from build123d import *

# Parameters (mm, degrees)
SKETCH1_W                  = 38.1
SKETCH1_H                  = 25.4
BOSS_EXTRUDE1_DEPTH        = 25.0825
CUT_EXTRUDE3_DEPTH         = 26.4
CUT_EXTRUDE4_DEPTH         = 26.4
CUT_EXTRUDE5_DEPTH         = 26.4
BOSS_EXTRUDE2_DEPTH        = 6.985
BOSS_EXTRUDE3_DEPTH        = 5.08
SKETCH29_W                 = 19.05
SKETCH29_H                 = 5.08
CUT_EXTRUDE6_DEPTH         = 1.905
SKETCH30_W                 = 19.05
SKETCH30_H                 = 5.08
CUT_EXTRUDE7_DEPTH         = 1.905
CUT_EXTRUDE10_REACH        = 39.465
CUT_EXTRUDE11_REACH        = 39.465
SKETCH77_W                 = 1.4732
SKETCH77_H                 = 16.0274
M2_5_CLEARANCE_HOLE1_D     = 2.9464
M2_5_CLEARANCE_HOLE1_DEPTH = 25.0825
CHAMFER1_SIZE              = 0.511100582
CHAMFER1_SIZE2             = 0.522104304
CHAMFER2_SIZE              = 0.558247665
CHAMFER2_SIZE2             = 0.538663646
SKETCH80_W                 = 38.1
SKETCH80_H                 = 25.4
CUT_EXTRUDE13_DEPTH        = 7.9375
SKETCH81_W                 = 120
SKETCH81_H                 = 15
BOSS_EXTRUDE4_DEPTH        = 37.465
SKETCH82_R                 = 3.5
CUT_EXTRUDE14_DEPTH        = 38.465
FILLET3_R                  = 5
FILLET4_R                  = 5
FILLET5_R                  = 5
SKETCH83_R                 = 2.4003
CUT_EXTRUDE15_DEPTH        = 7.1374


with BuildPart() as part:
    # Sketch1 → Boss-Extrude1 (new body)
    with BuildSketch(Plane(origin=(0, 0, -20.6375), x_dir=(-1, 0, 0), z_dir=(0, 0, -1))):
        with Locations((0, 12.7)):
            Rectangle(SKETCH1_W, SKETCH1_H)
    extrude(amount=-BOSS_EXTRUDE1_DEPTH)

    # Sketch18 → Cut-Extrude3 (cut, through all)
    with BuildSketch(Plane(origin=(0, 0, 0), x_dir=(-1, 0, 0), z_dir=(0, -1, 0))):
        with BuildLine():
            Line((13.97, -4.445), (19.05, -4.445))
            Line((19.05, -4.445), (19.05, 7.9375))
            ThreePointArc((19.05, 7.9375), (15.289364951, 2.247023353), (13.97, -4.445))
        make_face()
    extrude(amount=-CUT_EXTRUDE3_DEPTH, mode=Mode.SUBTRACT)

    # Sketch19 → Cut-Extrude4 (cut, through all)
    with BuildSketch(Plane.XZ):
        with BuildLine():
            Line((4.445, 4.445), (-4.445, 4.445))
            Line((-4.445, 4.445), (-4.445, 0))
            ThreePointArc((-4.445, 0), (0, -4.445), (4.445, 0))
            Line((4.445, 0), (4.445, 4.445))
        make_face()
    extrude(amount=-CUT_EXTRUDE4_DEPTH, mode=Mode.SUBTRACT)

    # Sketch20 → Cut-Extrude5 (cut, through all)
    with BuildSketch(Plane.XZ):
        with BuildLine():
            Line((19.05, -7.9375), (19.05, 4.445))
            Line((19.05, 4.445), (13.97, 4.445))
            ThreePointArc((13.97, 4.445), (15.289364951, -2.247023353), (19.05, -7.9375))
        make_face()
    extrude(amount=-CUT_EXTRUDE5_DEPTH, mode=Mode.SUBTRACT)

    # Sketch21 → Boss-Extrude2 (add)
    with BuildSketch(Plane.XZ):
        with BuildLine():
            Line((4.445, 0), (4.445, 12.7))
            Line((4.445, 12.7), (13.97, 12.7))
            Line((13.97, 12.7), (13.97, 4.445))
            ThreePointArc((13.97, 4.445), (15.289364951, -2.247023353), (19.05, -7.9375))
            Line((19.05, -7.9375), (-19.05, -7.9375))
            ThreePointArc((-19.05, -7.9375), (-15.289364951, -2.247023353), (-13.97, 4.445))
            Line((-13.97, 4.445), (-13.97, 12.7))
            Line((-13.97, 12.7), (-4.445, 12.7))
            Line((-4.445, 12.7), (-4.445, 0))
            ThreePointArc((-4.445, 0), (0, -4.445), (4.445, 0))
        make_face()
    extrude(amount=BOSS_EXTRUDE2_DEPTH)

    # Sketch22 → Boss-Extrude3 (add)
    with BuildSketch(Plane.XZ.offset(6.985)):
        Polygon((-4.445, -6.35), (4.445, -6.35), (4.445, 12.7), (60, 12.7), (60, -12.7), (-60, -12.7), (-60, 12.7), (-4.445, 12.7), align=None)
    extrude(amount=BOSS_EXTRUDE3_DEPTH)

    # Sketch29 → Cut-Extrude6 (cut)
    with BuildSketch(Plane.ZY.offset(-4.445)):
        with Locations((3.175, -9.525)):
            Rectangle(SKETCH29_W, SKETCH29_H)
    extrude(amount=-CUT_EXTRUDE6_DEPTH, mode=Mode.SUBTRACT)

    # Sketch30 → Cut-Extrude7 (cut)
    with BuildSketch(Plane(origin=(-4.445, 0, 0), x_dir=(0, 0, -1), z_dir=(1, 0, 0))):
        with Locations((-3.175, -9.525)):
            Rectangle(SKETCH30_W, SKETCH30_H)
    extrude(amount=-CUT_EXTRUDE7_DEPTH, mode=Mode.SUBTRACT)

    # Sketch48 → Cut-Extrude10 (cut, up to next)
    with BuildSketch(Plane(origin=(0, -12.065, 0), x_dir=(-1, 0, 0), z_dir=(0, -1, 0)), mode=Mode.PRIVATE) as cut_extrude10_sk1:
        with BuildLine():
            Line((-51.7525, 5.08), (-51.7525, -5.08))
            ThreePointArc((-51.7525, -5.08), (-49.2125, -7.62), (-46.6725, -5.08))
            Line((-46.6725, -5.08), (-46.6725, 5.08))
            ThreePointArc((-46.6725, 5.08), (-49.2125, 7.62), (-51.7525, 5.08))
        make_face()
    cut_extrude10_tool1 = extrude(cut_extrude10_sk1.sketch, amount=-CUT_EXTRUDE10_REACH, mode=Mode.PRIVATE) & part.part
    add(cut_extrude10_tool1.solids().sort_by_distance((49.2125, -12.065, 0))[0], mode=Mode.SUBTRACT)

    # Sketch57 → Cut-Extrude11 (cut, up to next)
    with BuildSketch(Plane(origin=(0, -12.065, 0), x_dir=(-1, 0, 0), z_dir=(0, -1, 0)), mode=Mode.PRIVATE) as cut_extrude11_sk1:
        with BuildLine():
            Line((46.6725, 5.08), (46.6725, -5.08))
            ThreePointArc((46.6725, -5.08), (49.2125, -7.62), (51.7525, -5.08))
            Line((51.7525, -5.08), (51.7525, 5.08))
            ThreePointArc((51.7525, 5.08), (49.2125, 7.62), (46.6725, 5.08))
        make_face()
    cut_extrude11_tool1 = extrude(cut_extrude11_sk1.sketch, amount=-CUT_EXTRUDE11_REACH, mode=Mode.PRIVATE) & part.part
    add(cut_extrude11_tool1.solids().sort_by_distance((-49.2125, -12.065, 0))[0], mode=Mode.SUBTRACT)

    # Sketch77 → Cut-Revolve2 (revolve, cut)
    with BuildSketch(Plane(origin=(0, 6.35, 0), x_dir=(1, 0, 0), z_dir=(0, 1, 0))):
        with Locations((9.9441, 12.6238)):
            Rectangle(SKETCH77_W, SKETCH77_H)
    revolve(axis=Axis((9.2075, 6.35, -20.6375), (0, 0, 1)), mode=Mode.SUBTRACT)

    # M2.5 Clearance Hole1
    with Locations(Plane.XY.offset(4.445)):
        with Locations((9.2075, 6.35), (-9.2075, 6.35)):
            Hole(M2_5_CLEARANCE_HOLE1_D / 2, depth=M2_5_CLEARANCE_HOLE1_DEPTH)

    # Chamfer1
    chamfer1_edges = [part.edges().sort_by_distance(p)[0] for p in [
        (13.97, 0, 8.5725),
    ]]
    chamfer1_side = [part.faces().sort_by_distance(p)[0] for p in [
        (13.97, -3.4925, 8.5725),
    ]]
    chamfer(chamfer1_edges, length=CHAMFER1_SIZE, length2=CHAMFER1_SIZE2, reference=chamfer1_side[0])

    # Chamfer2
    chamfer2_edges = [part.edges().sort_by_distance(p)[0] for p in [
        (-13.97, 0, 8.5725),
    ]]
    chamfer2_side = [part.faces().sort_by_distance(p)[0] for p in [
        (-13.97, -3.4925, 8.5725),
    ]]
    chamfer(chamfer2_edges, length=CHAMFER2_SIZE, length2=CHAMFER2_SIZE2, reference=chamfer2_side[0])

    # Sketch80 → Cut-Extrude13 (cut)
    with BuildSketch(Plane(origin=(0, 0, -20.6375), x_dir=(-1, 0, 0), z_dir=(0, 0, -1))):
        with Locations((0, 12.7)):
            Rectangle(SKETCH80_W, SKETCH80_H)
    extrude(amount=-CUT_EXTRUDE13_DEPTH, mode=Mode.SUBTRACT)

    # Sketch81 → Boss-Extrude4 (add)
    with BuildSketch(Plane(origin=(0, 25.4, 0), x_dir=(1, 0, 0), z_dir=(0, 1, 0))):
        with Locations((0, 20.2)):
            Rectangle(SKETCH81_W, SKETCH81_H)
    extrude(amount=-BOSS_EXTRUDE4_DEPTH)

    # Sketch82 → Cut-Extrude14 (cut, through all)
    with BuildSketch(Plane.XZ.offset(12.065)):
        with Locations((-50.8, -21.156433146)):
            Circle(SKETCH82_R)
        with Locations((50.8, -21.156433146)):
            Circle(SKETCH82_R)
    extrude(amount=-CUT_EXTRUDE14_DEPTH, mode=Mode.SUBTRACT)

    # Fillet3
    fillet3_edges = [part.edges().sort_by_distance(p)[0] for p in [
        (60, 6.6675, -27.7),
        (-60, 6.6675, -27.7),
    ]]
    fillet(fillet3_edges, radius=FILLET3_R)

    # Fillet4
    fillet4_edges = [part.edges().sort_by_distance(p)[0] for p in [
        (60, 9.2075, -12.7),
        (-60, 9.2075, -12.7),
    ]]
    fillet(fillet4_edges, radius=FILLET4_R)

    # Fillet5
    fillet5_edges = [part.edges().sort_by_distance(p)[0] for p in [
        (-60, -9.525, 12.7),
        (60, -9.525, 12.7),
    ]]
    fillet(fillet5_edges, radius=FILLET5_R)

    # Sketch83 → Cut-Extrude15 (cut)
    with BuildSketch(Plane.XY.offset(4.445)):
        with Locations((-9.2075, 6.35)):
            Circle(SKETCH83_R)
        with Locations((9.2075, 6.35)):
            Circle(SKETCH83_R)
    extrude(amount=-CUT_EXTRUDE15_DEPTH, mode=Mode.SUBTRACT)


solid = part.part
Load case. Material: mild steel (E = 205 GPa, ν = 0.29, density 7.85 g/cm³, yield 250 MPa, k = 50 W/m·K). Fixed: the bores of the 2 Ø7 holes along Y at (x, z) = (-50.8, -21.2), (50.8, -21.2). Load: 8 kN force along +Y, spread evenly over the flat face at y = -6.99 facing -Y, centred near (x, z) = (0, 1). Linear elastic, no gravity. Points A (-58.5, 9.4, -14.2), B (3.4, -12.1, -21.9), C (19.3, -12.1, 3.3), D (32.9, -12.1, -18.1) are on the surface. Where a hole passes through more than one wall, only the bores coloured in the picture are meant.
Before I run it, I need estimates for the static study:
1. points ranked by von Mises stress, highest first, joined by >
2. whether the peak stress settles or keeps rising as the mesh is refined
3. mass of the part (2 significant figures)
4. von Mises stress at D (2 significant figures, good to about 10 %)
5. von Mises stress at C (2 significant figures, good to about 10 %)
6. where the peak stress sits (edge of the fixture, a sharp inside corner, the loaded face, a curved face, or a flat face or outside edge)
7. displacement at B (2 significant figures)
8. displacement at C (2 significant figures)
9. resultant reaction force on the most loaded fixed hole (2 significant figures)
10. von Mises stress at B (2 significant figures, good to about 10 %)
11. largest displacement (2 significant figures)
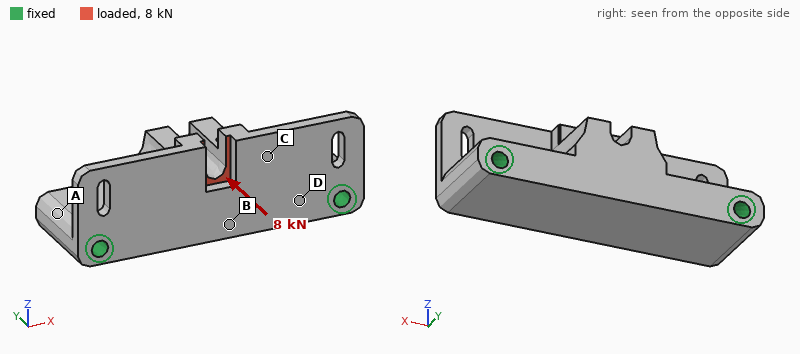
D > B > C > A
keeps rising
730 g
44 MPa
14 MPa
edge of the fixture
14 µm
27 µm
4.0 kN
27 MPa
43 µm
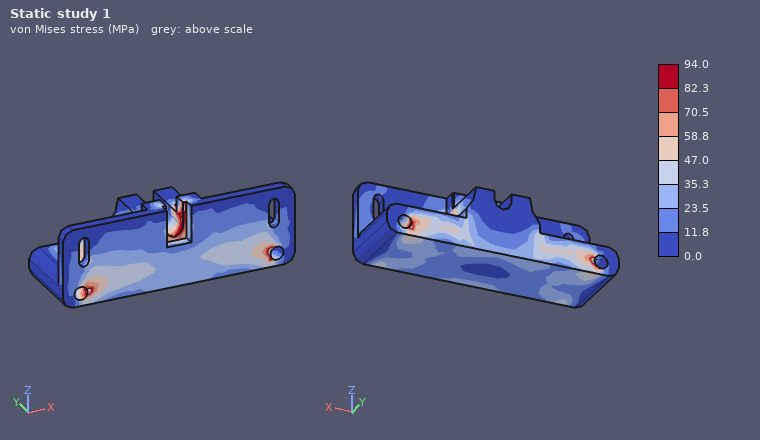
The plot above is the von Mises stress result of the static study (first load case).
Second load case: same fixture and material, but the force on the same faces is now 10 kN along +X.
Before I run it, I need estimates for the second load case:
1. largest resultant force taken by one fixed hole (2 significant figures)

5.6 kN
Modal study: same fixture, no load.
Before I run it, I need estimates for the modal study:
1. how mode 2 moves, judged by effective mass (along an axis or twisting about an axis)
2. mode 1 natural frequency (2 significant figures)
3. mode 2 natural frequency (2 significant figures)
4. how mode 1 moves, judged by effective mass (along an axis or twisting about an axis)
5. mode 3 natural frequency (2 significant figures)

along Z
5800 Hz
6300 Hz
along Y
6900 Hz
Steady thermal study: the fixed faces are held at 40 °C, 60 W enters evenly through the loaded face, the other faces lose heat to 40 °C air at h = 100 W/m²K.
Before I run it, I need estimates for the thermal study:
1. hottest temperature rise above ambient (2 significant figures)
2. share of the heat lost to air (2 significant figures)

70 K
50 %
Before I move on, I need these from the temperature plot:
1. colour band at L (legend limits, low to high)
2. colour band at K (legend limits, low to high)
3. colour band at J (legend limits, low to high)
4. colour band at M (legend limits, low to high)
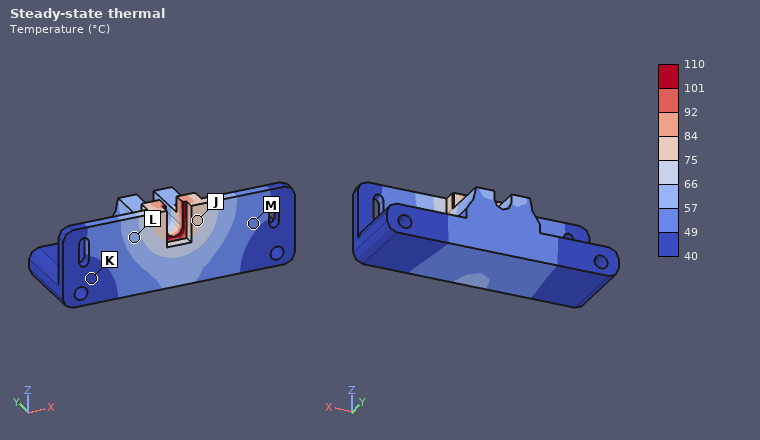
57 to 66 °C
40 to 49 °C
75 to 84 °C
49 to 57 °C
